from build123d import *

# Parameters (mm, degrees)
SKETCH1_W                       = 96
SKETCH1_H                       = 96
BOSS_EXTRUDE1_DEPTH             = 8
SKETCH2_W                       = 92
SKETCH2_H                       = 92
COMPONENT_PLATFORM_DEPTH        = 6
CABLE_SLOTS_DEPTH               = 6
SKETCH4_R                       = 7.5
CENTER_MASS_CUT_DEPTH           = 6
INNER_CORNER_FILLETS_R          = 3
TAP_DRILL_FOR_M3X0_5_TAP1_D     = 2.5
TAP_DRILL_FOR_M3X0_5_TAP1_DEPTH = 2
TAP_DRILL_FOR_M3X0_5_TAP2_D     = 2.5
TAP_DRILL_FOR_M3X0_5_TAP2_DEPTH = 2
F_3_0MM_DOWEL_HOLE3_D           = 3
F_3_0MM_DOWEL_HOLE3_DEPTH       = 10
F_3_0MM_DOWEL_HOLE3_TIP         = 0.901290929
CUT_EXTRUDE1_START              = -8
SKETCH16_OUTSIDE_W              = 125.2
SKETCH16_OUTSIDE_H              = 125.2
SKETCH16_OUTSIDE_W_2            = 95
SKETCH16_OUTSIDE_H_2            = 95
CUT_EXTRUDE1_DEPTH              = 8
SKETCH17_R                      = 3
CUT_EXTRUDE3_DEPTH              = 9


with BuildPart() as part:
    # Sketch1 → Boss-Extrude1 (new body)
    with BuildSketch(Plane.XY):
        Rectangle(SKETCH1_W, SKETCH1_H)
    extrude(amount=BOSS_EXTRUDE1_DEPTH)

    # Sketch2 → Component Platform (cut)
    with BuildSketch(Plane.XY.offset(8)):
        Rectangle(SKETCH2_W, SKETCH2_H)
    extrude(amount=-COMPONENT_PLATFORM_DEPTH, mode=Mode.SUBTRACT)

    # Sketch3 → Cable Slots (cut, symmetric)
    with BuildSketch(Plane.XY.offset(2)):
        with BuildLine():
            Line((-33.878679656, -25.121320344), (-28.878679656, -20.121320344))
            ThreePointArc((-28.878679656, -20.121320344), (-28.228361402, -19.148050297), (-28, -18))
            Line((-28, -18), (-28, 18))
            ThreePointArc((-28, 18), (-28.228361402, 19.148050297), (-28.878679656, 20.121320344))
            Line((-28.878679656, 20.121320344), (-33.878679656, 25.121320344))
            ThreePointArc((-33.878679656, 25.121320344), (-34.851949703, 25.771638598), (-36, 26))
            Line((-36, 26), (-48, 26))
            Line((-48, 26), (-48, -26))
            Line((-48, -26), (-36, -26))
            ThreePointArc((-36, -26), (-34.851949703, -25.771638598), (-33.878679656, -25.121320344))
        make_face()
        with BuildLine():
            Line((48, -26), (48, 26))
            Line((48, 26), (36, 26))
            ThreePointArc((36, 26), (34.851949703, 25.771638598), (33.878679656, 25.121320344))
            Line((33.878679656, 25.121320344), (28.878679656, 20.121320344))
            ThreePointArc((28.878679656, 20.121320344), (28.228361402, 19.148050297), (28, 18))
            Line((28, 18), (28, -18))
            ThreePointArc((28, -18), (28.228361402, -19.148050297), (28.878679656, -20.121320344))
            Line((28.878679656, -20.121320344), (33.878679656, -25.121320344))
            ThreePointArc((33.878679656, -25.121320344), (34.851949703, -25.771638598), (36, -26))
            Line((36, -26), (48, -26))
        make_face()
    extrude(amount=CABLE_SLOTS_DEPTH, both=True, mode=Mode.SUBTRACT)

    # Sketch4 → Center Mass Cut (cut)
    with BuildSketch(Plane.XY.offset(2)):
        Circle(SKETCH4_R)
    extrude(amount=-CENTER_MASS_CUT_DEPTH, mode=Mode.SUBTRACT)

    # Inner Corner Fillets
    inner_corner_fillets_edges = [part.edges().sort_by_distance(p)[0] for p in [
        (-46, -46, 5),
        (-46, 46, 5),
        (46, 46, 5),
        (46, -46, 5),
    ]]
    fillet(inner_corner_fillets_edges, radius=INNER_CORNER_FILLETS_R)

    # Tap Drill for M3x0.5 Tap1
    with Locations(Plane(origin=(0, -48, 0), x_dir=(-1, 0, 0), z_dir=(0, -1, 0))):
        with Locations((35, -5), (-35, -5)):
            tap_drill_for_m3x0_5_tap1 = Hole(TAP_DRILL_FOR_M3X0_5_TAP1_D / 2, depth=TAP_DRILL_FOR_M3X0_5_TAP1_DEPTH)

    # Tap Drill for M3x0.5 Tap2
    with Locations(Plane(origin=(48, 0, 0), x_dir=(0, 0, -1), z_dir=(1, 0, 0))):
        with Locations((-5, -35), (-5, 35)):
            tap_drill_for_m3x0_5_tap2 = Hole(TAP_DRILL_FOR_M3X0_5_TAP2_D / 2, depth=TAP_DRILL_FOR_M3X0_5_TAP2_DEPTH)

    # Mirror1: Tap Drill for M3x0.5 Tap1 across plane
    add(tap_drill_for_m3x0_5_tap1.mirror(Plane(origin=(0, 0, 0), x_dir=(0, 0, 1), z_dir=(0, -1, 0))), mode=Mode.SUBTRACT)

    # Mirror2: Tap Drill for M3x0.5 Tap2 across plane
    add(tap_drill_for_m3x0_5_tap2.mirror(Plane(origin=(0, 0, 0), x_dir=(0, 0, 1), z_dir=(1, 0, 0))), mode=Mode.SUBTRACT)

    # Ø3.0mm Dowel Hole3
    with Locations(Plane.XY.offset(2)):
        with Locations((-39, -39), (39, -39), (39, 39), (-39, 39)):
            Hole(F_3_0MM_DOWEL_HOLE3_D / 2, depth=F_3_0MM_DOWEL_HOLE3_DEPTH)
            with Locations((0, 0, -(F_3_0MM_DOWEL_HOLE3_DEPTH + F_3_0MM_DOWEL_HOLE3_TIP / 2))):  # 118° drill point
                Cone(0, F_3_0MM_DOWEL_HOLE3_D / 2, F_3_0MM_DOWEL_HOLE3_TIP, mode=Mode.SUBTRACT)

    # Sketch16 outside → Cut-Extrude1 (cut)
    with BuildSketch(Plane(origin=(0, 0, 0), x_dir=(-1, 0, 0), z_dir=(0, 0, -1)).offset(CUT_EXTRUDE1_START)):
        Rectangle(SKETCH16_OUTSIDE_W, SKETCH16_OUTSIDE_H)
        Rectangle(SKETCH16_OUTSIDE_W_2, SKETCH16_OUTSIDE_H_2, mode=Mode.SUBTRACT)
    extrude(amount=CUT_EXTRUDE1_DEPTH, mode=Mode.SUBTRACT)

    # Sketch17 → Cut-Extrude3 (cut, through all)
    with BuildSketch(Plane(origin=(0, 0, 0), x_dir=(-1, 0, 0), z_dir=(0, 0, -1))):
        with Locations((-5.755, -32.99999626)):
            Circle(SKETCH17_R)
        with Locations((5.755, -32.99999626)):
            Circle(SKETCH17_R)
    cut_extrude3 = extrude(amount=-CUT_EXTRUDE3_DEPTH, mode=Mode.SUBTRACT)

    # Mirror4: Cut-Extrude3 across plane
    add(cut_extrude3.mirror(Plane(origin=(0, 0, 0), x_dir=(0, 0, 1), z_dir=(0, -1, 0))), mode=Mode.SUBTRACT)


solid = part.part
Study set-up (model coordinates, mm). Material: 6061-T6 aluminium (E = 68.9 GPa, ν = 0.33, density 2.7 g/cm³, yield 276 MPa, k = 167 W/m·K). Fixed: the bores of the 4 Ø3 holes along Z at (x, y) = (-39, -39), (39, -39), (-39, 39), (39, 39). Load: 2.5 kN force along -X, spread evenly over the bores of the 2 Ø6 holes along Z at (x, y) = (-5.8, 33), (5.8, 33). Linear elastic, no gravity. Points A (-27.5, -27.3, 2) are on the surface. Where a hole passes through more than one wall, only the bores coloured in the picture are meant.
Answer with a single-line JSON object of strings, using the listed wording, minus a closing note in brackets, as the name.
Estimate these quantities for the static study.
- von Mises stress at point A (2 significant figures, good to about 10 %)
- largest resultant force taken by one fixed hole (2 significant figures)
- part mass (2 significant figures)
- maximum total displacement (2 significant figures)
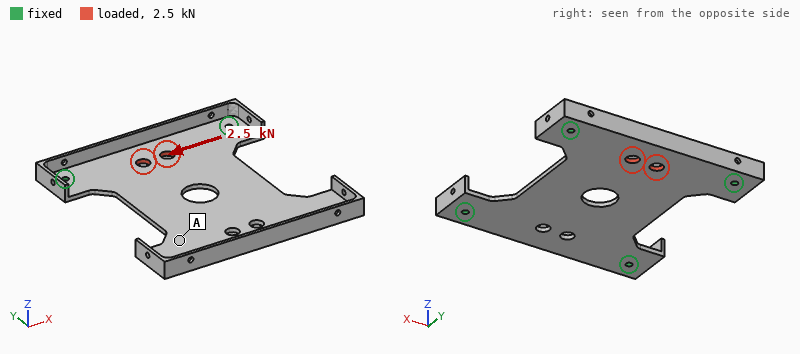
{"von Mises stress at point A": "6.8 MPa", "largest resultant force taken by one fixed hole": "1.1 kN", "part mass": "43 g", "maximum total displacement": "22 µm"}
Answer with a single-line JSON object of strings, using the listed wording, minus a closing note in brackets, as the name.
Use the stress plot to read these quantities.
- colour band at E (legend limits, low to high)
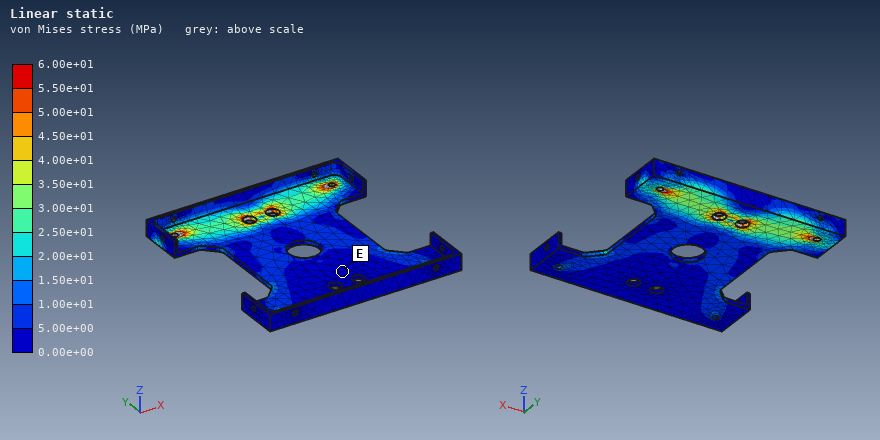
{"colour band at E": "0.00e+00 to 5.00e+00 MPa"}
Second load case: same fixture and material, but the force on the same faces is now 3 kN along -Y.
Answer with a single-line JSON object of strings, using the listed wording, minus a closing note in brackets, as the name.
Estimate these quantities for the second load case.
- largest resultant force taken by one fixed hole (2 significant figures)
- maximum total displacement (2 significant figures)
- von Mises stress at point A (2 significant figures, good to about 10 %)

{"largest resultant force taken by one fixed hole": "930 N", "maximum total displacement": "68 µm", "von Mises stress at point A": "29 MPa"}
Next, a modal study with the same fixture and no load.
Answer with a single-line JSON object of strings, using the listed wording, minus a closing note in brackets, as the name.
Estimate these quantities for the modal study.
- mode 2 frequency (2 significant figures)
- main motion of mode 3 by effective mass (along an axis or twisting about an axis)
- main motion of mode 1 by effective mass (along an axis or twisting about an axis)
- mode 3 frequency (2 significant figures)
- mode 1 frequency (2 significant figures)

{"mode 2 frequency": "2400 Hz", "main motion of mode 3 by effective mass": "twisting about X", "main motion of mode 1 by effective mass": "along Z", "mode 3 frequency": "2500 Hz", "mode 1 frequency": "1200 Hz"}
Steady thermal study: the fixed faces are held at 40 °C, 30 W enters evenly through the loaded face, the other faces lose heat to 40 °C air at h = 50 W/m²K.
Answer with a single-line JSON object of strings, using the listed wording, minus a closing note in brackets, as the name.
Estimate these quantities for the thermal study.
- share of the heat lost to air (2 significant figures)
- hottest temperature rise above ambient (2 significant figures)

{"share of the heat lost to air": "34 %", "hottest temperature rise above ambient": "46 K"}
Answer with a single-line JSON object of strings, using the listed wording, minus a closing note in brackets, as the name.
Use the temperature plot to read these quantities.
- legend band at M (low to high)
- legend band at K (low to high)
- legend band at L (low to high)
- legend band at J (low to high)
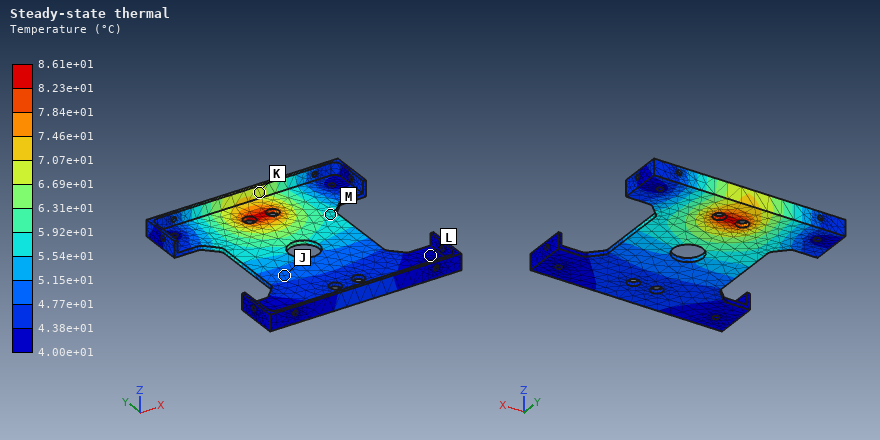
{"legend band at M": "5.54e+01 to 5.92e+01 °C", "legend band at K": "6.69e+01 to 7.07e+01 °C", "legend band at L": "4.00e+01 to 4.38e+01 °C", "legend band at J": "4.77e+01 to 5.15e+01 °C"}
